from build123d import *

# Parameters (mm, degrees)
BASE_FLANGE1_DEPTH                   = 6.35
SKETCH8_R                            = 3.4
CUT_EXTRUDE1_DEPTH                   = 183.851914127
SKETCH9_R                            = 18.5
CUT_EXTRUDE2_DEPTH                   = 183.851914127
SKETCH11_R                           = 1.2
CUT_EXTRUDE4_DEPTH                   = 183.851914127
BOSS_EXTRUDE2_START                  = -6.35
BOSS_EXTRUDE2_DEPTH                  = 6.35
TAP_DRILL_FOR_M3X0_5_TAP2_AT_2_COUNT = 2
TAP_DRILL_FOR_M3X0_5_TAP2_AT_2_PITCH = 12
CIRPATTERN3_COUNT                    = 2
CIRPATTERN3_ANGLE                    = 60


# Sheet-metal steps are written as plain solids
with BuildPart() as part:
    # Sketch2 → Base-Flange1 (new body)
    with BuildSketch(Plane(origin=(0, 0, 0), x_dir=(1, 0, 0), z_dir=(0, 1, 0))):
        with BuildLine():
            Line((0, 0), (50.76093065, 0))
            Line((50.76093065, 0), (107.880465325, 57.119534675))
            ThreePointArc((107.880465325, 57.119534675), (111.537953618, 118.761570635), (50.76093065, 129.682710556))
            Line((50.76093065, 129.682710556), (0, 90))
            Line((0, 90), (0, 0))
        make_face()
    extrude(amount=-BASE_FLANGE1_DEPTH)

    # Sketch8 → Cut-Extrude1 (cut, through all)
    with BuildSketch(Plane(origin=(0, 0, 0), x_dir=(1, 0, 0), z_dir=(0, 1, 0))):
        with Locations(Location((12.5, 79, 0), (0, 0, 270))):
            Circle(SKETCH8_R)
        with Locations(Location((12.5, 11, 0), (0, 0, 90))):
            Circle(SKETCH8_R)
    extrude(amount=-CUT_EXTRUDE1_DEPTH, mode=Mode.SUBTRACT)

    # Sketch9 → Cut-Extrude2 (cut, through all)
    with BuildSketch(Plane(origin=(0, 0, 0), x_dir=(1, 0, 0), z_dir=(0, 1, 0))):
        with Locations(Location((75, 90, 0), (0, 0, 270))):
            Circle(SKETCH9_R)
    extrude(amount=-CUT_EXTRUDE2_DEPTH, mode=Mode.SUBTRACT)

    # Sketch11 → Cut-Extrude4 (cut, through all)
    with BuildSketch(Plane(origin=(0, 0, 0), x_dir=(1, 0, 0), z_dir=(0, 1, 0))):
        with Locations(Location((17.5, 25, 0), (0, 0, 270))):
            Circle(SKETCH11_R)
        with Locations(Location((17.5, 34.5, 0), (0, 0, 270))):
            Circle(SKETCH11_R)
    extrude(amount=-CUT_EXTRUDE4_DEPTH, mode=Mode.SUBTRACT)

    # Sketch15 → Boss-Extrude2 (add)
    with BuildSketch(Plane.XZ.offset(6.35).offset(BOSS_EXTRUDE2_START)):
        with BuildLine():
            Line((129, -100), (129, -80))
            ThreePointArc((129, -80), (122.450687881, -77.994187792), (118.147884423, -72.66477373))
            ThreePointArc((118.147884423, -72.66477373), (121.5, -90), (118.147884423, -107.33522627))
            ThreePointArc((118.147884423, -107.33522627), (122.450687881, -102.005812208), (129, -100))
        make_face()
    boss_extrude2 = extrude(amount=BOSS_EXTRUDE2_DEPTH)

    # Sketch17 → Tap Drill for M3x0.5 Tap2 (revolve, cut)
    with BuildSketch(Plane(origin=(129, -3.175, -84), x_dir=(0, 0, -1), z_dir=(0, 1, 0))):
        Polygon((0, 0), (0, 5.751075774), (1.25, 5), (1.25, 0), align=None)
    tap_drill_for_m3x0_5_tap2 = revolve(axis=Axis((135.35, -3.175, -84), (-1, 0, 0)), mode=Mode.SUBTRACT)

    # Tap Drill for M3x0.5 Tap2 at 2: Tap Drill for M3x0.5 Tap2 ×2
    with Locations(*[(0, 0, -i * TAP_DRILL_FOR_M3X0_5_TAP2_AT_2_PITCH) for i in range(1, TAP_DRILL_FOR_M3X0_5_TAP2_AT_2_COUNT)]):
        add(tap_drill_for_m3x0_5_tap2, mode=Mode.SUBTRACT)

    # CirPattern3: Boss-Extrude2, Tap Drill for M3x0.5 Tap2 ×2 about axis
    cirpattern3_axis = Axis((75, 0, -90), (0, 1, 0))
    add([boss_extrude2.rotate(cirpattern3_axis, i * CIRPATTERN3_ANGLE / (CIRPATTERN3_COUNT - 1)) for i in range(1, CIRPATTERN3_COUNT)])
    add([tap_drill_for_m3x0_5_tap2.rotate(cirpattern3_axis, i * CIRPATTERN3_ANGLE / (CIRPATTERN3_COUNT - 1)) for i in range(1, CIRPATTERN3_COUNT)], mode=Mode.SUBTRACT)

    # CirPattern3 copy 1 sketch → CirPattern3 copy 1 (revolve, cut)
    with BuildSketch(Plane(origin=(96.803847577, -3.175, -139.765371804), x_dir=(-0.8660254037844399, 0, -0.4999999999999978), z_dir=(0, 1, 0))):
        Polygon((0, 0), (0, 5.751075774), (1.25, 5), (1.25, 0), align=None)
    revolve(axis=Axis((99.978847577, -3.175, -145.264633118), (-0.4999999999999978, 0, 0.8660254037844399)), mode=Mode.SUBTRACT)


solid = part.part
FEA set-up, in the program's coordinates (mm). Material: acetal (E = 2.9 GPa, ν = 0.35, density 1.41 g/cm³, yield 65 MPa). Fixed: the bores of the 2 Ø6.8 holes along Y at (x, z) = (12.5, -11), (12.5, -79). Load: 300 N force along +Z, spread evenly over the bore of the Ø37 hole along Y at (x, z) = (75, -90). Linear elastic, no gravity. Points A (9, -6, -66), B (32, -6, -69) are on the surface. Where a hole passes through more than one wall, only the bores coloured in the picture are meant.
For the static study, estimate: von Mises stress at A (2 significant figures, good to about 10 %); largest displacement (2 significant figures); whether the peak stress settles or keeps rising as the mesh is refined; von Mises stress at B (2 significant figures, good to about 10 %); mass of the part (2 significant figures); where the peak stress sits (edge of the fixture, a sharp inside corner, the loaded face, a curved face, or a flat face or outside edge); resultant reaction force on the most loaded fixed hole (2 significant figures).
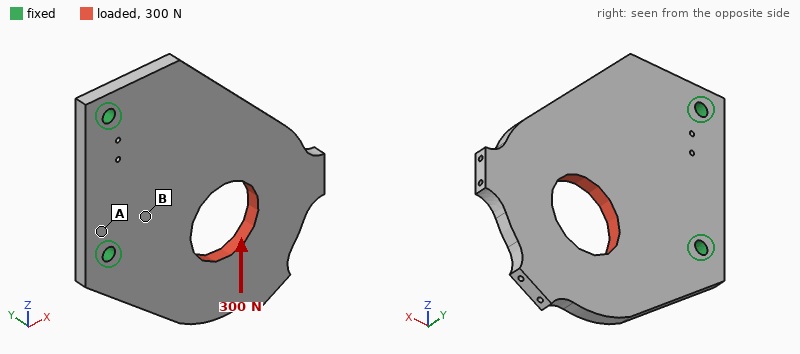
0.65 MPa
0.13 mm
keeps rising
1.5 MPa
100 g
edge of the fixture
310 N
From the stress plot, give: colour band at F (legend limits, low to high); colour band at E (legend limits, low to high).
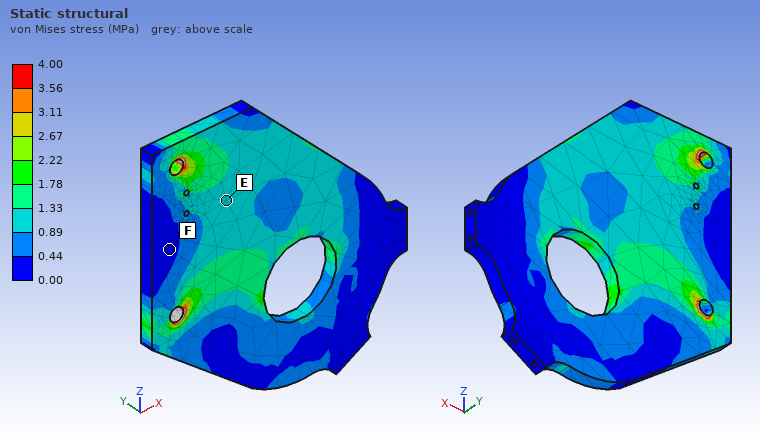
0.00 to 0.44 MPa
0.89 to 1.33 MPa
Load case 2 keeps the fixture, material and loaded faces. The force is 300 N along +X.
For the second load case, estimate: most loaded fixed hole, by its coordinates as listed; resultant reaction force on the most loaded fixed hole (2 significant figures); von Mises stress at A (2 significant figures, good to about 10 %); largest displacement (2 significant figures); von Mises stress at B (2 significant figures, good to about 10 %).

(12.5, -79)
340 N
0.61 MPa
84 µm
1.2 MPa
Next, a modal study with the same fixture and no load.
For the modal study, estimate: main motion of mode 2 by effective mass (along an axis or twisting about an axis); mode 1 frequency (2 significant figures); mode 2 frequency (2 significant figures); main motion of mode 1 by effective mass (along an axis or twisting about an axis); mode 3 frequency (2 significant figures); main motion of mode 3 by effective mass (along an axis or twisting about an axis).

twisting about X
120 Hz
300 Hz
along Y
580 Hz
along Y
